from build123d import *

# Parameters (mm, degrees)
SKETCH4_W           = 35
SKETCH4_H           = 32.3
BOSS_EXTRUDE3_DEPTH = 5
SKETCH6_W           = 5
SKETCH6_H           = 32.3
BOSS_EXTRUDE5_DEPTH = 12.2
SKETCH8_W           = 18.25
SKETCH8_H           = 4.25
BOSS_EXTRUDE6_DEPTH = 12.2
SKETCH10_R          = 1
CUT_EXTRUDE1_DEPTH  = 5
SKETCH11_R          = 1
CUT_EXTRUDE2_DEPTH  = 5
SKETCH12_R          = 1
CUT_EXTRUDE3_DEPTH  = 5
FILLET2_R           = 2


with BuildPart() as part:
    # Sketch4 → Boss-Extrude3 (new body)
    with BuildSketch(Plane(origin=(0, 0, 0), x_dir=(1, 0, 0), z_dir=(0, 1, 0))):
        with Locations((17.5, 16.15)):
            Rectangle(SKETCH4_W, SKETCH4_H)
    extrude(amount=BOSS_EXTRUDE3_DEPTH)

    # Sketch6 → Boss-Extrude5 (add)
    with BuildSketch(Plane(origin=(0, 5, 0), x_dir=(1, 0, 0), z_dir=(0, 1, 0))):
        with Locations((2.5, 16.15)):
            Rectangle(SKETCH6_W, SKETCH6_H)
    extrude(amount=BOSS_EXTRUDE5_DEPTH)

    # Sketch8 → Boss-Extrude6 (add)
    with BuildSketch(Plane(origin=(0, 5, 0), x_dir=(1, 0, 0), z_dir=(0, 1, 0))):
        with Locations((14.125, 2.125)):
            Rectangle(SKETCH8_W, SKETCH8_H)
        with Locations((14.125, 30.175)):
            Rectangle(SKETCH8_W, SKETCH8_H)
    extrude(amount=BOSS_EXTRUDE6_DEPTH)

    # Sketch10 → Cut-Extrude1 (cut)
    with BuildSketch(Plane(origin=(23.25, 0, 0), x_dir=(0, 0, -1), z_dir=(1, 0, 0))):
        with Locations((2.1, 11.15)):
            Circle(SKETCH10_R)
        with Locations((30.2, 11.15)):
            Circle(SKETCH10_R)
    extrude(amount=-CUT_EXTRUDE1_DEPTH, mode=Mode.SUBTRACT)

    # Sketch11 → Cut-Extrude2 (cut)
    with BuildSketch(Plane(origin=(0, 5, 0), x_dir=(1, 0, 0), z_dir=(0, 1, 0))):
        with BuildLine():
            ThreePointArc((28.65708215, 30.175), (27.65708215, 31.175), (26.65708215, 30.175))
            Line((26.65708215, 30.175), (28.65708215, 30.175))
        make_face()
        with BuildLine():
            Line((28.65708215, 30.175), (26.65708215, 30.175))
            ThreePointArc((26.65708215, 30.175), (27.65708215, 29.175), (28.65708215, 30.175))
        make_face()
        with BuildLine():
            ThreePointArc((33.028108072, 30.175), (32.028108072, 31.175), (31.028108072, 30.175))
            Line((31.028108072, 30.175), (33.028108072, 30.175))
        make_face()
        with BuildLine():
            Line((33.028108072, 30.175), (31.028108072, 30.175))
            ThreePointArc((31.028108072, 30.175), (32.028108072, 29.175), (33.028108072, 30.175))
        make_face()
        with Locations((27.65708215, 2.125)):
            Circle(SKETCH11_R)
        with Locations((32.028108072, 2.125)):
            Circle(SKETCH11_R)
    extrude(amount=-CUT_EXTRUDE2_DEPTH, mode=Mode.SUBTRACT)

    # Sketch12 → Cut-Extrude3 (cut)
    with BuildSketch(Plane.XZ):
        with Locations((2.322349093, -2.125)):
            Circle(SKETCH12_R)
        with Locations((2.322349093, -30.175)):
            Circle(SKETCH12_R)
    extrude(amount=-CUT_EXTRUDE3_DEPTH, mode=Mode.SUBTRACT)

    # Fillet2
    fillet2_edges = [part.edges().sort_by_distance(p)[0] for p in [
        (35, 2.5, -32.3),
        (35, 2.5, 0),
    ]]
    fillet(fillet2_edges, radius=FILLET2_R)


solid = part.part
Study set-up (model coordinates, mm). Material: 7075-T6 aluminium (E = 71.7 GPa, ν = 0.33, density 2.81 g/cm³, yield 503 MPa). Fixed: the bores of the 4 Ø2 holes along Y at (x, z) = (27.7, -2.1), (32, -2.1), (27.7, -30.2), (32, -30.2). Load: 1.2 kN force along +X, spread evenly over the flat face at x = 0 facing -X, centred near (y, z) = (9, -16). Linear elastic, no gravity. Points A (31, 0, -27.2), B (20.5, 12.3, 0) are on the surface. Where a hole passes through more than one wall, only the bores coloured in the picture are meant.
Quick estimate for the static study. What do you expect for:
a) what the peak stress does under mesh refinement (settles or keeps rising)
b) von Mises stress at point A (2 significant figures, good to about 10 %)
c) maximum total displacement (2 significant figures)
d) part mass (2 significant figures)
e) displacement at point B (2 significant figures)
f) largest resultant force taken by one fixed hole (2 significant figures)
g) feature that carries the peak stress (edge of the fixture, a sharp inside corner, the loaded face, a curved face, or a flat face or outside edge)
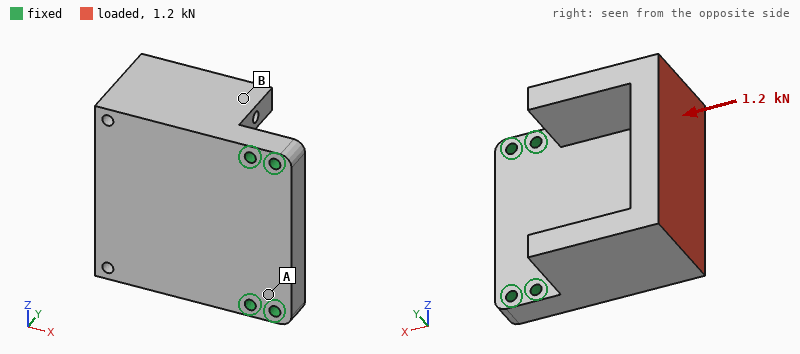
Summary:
keeps rising
23 MPa
0.11 mm
26 g
0.040 mm
530 N
edge of the fixture
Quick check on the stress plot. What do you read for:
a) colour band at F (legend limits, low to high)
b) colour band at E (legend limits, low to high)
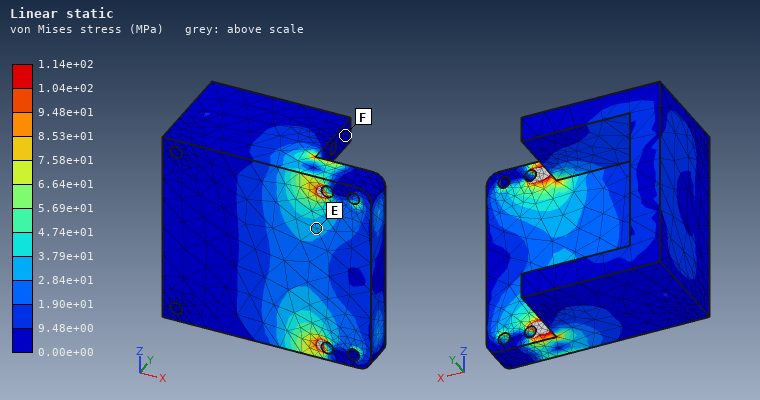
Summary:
0.00e+00 to 9.48e+00 MPa
2.84e+01 to 3.79e+01 MPa
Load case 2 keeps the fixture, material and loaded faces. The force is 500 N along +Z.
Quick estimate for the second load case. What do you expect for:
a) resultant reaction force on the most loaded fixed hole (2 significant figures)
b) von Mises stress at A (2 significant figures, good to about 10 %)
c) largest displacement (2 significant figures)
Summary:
480 N
5.8 MPa
20 µm
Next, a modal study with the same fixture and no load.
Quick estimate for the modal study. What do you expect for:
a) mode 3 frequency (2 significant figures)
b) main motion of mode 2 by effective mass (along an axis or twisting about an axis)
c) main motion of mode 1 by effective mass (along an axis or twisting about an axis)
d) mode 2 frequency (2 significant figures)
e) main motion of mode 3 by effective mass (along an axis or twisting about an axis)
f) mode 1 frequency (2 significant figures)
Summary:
13 kHz
along Z
along Y
6400 Hz
along Z
2800 Hz
